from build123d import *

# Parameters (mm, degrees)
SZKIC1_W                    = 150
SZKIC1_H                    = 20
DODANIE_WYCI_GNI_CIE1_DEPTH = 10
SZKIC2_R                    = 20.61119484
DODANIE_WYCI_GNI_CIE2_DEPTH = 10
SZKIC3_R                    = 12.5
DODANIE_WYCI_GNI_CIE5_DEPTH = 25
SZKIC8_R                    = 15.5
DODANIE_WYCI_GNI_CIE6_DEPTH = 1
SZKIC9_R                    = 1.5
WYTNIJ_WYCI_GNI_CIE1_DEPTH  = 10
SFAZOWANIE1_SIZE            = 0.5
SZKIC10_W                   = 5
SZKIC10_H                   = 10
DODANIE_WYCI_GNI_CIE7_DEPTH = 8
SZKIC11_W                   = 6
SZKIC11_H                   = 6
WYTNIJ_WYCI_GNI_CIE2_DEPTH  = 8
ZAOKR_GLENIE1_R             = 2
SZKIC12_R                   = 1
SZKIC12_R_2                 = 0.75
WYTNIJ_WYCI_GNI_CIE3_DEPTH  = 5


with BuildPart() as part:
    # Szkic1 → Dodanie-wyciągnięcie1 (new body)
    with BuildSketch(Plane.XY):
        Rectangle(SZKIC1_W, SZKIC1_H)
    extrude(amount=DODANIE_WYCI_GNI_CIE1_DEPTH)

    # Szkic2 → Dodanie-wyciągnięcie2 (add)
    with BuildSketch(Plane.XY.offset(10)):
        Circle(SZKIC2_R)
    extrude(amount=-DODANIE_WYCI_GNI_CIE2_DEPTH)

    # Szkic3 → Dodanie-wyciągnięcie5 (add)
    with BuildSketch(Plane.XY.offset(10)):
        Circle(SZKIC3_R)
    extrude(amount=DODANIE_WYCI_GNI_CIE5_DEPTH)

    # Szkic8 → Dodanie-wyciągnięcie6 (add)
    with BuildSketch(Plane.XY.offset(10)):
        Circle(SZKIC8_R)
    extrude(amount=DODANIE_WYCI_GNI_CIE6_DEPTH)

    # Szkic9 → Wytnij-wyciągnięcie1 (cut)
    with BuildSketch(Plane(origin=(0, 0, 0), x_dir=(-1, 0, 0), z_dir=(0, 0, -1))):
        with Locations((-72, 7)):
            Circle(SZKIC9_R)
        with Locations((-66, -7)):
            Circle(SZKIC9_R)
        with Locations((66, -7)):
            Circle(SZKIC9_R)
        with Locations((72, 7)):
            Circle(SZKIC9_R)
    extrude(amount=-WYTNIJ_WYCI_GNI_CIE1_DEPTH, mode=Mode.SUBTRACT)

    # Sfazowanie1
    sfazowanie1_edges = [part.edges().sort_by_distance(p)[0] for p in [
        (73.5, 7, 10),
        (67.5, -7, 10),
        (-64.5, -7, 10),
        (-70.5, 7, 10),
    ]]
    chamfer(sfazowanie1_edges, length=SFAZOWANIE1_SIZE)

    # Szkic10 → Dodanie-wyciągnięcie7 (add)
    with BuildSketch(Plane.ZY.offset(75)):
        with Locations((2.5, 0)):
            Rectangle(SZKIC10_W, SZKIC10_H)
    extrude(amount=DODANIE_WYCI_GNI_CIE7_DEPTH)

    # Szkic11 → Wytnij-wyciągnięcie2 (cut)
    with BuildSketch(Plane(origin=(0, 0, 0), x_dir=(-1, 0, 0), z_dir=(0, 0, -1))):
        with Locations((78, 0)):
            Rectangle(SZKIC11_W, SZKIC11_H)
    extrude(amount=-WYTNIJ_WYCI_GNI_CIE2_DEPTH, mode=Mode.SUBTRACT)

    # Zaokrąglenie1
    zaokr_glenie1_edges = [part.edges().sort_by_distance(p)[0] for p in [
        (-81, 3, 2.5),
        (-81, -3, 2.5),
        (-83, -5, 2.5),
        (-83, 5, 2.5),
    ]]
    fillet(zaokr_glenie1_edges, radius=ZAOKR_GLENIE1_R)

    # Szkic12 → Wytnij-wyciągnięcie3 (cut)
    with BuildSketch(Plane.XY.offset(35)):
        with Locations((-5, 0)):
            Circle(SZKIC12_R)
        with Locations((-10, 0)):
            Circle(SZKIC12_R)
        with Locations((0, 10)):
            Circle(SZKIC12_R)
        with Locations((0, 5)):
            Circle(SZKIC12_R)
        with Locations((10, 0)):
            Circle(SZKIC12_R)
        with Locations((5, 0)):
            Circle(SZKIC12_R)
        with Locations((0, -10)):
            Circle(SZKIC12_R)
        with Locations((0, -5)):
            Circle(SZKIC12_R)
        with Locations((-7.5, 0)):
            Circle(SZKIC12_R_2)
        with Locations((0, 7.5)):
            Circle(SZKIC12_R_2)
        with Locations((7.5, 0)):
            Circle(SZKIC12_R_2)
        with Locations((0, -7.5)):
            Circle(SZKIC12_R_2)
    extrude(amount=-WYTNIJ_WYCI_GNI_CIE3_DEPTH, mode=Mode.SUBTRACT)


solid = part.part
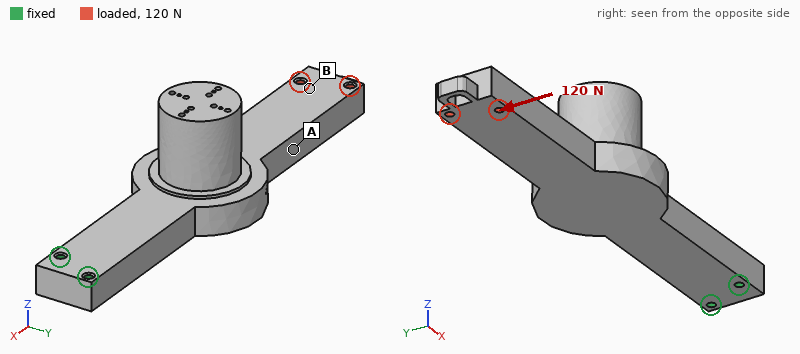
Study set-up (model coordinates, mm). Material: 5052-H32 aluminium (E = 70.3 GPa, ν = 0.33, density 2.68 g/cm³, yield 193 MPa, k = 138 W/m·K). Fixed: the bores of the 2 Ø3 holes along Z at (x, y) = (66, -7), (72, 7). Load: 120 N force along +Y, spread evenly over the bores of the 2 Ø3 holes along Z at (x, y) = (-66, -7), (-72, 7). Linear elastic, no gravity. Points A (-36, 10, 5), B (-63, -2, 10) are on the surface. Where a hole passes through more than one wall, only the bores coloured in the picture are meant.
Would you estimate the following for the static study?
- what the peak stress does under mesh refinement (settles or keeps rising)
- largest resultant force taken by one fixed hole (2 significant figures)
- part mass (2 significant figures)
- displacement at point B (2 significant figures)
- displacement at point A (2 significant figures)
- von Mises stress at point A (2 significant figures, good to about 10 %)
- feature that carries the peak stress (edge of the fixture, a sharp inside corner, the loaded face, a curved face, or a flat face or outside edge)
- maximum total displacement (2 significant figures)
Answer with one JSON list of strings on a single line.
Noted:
["keeps rising", "1.1 kN", "130 g", "0.18 mm", "0.13 mm", "5.9 MPa", "edge of the fixture", "0.22 mm"]
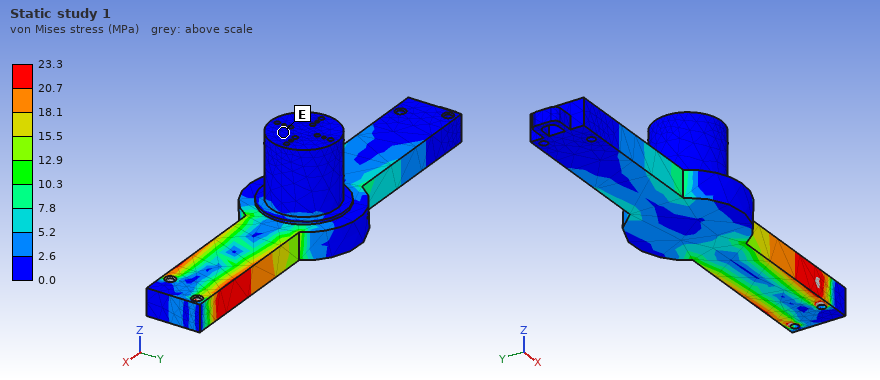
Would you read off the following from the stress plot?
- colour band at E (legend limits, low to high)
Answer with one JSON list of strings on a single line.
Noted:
["0.0 to 2.6 MPa"]
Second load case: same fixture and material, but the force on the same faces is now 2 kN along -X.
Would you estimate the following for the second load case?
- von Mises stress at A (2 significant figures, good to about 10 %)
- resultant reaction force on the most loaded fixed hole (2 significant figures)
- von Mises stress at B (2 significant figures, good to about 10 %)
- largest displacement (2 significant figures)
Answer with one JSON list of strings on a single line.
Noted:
["9.8 MPa", "1.0 kN", "5.7 MPa", "61 µm"]
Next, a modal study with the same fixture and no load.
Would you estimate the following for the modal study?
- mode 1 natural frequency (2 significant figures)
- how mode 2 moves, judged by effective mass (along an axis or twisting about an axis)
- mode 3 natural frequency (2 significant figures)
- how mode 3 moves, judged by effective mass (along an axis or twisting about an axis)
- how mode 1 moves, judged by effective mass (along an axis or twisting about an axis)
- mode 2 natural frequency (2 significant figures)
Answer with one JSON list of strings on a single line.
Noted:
["360 Hz", "along Y", "1800 Hz", "twisting about X", "along Z", "720 Hz"]
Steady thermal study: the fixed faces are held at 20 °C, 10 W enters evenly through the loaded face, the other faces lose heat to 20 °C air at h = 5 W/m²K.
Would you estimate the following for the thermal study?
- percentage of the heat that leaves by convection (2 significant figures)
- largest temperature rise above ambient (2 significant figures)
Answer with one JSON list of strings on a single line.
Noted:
["13 %", "42 K"]
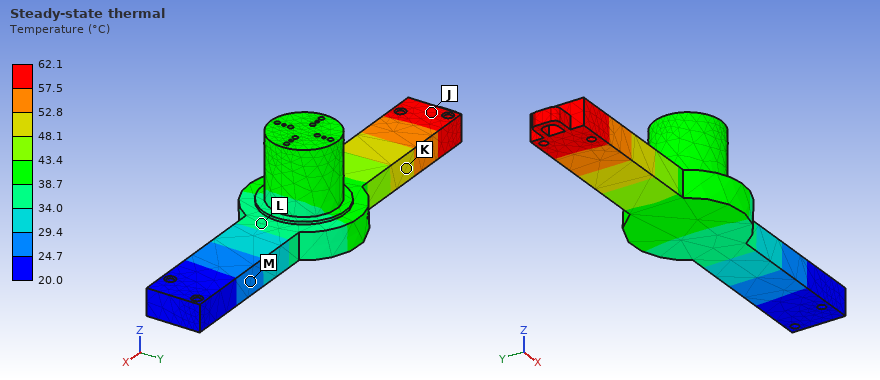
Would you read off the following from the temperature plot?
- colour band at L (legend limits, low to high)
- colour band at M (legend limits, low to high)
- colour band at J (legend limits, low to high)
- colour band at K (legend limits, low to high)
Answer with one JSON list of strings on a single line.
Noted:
["34.0 to 38.7 °C", "24.7 to 29.4 °C", "57.5 to 62.1 °C", "48.1 to 52.8 °C"]
